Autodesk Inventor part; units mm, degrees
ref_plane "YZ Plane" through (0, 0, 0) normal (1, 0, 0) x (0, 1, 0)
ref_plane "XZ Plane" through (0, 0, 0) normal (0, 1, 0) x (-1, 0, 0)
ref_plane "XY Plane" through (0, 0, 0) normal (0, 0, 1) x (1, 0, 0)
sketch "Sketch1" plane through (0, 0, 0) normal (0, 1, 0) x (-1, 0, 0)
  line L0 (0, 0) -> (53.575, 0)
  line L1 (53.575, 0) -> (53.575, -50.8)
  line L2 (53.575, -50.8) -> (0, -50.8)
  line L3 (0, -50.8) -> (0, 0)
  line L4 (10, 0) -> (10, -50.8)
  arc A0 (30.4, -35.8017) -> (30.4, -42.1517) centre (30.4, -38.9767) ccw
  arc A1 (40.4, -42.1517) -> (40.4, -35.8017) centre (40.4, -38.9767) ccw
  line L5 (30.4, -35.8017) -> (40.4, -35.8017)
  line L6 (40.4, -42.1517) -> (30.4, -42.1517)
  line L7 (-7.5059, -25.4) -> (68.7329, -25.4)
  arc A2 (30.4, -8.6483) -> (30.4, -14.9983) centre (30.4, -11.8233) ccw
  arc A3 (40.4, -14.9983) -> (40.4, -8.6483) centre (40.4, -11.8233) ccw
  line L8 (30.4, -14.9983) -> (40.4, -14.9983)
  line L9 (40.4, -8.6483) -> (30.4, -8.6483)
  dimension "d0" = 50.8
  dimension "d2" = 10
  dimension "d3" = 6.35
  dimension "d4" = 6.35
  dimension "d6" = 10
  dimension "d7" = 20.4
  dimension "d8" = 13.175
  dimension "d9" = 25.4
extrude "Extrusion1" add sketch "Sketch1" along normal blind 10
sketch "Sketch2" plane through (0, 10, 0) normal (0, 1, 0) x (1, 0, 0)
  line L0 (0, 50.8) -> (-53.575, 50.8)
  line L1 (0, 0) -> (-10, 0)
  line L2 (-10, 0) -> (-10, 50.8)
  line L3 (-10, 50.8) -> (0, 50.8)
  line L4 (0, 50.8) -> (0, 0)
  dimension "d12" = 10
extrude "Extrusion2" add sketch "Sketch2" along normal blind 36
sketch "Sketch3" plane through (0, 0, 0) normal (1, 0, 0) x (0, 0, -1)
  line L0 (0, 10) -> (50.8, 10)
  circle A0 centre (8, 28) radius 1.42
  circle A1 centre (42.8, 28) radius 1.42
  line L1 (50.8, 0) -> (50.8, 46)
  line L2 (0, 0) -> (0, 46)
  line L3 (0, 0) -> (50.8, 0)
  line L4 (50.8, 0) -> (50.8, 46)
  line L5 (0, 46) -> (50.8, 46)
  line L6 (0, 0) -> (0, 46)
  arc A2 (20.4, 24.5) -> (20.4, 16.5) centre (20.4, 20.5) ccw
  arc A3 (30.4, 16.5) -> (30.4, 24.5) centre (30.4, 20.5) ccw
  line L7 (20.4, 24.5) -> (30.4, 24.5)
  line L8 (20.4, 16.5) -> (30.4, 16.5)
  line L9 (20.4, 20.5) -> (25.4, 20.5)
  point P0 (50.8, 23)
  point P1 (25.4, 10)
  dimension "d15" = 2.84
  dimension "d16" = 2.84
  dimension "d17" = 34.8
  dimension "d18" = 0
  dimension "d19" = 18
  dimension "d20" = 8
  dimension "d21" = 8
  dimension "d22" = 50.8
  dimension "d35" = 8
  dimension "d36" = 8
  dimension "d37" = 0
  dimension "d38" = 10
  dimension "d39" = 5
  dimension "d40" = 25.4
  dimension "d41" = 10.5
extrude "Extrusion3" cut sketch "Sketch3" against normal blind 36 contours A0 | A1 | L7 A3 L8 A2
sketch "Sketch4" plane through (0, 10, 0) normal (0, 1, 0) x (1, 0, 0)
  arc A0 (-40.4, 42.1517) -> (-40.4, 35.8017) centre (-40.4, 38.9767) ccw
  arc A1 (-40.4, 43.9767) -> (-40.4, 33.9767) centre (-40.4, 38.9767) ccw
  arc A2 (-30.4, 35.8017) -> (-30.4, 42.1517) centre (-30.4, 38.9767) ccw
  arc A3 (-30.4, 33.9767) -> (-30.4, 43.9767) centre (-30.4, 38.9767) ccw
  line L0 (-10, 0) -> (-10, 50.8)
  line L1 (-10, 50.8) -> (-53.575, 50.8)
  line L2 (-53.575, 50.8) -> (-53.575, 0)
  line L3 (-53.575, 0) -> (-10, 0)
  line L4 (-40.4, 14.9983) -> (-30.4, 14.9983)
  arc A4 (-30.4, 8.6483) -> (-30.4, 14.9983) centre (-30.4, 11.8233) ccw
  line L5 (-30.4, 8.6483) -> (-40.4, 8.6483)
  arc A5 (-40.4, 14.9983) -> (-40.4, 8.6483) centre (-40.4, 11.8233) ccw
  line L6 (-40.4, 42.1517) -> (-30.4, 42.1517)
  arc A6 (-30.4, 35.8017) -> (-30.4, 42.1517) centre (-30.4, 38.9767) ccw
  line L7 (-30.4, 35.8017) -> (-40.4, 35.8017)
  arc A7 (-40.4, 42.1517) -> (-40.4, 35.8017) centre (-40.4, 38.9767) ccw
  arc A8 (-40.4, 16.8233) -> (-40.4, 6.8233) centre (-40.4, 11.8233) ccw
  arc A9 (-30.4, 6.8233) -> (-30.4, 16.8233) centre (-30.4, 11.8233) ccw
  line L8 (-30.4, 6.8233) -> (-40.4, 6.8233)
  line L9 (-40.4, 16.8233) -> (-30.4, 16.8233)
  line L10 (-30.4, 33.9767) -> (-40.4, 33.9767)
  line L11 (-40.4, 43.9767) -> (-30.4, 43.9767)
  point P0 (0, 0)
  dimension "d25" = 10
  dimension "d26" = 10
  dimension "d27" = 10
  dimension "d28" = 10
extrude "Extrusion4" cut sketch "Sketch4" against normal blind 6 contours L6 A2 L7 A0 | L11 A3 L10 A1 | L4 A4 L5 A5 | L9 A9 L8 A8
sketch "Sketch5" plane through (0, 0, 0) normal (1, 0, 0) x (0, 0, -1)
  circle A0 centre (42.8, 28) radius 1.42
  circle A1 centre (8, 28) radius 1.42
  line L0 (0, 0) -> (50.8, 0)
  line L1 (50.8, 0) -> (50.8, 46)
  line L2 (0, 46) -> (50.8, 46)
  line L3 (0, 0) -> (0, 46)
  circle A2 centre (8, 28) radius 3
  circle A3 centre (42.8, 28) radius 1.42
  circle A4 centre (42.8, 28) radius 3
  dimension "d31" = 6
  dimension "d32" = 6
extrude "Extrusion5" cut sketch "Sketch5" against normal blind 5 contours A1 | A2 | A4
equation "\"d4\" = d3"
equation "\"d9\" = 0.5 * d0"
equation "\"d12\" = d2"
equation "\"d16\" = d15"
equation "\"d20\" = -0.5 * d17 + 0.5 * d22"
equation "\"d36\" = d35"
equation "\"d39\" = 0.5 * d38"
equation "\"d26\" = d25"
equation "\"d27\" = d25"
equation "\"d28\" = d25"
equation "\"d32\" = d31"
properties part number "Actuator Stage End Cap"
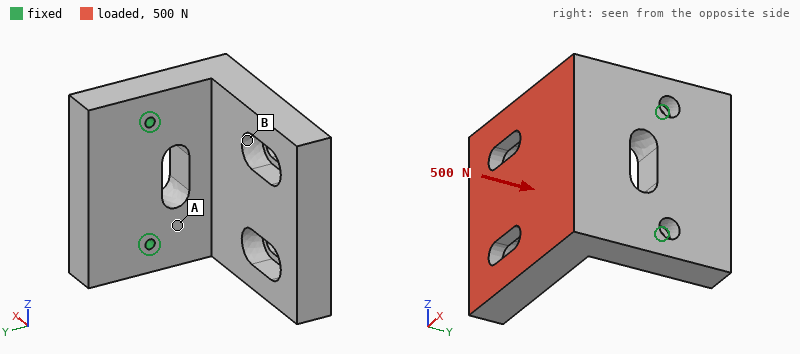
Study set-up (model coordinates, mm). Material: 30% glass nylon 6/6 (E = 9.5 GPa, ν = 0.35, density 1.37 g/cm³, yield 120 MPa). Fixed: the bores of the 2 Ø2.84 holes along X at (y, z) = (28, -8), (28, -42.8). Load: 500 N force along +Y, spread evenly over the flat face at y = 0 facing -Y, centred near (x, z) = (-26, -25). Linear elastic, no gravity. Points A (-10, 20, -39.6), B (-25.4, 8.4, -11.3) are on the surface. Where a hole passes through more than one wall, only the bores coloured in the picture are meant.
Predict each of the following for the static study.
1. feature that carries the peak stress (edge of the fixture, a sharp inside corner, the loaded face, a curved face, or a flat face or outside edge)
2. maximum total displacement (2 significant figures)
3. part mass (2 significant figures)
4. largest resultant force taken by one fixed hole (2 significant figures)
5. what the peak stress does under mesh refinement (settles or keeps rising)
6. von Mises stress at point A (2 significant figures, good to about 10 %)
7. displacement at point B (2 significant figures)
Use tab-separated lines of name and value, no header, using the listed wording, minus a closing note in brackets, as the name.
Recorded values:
feature that carries the peak stress	edge of the fixture
maximum total displacement	0.93 mm
part mass	56 g
largest resultant force taken by one fixed hole	260 N
what the peak stress does under mesh refinement	keeps rising
von Mises stress at point A	20 MPa
displacement at point B	0.38 mm
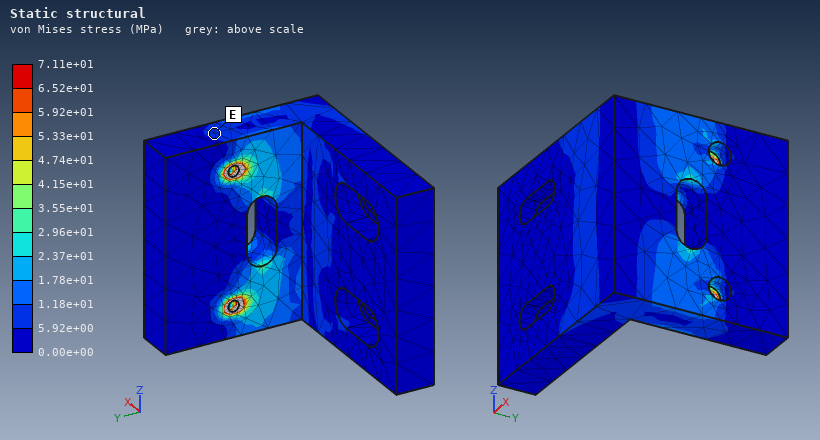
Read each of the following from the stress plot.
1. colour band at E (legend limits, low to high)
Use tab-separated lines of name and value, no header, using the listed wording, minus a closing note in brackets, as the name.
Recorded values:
colour band at E	5.92e+00 to 1.18e+01 MPa
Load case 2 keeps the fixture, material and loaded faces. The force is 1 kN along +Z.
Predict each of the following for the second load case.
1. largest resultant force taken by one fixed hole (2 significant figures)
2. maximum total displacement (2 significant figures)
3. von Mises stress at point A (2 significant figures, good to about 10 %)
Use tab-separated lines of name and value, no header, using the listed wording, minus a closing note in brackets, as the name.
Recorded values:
largest resultant force taken by one fixed hole	1.0 kN
maximum total displacement	0.38 mm
von Mises stress at point A	26 MPa
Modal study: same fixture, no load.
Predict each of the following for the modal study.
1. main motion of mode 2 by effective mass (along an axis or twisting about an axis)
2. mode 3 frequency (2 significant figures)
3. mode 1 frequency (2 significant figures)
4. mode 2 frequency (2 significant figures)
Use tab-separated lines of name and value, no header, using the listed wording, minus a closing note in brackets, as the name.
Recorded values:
main motion of mode 2 by effective mass	along Z
mode 3 frequency	2300 Hz
mode 1 frequency	670 Hz
mode 2 frequency	1600 Hz
